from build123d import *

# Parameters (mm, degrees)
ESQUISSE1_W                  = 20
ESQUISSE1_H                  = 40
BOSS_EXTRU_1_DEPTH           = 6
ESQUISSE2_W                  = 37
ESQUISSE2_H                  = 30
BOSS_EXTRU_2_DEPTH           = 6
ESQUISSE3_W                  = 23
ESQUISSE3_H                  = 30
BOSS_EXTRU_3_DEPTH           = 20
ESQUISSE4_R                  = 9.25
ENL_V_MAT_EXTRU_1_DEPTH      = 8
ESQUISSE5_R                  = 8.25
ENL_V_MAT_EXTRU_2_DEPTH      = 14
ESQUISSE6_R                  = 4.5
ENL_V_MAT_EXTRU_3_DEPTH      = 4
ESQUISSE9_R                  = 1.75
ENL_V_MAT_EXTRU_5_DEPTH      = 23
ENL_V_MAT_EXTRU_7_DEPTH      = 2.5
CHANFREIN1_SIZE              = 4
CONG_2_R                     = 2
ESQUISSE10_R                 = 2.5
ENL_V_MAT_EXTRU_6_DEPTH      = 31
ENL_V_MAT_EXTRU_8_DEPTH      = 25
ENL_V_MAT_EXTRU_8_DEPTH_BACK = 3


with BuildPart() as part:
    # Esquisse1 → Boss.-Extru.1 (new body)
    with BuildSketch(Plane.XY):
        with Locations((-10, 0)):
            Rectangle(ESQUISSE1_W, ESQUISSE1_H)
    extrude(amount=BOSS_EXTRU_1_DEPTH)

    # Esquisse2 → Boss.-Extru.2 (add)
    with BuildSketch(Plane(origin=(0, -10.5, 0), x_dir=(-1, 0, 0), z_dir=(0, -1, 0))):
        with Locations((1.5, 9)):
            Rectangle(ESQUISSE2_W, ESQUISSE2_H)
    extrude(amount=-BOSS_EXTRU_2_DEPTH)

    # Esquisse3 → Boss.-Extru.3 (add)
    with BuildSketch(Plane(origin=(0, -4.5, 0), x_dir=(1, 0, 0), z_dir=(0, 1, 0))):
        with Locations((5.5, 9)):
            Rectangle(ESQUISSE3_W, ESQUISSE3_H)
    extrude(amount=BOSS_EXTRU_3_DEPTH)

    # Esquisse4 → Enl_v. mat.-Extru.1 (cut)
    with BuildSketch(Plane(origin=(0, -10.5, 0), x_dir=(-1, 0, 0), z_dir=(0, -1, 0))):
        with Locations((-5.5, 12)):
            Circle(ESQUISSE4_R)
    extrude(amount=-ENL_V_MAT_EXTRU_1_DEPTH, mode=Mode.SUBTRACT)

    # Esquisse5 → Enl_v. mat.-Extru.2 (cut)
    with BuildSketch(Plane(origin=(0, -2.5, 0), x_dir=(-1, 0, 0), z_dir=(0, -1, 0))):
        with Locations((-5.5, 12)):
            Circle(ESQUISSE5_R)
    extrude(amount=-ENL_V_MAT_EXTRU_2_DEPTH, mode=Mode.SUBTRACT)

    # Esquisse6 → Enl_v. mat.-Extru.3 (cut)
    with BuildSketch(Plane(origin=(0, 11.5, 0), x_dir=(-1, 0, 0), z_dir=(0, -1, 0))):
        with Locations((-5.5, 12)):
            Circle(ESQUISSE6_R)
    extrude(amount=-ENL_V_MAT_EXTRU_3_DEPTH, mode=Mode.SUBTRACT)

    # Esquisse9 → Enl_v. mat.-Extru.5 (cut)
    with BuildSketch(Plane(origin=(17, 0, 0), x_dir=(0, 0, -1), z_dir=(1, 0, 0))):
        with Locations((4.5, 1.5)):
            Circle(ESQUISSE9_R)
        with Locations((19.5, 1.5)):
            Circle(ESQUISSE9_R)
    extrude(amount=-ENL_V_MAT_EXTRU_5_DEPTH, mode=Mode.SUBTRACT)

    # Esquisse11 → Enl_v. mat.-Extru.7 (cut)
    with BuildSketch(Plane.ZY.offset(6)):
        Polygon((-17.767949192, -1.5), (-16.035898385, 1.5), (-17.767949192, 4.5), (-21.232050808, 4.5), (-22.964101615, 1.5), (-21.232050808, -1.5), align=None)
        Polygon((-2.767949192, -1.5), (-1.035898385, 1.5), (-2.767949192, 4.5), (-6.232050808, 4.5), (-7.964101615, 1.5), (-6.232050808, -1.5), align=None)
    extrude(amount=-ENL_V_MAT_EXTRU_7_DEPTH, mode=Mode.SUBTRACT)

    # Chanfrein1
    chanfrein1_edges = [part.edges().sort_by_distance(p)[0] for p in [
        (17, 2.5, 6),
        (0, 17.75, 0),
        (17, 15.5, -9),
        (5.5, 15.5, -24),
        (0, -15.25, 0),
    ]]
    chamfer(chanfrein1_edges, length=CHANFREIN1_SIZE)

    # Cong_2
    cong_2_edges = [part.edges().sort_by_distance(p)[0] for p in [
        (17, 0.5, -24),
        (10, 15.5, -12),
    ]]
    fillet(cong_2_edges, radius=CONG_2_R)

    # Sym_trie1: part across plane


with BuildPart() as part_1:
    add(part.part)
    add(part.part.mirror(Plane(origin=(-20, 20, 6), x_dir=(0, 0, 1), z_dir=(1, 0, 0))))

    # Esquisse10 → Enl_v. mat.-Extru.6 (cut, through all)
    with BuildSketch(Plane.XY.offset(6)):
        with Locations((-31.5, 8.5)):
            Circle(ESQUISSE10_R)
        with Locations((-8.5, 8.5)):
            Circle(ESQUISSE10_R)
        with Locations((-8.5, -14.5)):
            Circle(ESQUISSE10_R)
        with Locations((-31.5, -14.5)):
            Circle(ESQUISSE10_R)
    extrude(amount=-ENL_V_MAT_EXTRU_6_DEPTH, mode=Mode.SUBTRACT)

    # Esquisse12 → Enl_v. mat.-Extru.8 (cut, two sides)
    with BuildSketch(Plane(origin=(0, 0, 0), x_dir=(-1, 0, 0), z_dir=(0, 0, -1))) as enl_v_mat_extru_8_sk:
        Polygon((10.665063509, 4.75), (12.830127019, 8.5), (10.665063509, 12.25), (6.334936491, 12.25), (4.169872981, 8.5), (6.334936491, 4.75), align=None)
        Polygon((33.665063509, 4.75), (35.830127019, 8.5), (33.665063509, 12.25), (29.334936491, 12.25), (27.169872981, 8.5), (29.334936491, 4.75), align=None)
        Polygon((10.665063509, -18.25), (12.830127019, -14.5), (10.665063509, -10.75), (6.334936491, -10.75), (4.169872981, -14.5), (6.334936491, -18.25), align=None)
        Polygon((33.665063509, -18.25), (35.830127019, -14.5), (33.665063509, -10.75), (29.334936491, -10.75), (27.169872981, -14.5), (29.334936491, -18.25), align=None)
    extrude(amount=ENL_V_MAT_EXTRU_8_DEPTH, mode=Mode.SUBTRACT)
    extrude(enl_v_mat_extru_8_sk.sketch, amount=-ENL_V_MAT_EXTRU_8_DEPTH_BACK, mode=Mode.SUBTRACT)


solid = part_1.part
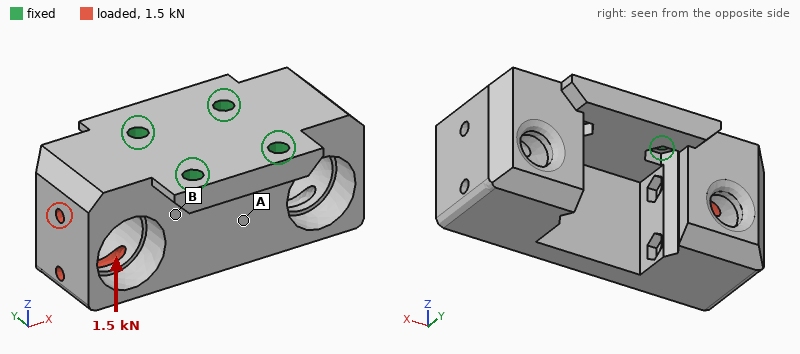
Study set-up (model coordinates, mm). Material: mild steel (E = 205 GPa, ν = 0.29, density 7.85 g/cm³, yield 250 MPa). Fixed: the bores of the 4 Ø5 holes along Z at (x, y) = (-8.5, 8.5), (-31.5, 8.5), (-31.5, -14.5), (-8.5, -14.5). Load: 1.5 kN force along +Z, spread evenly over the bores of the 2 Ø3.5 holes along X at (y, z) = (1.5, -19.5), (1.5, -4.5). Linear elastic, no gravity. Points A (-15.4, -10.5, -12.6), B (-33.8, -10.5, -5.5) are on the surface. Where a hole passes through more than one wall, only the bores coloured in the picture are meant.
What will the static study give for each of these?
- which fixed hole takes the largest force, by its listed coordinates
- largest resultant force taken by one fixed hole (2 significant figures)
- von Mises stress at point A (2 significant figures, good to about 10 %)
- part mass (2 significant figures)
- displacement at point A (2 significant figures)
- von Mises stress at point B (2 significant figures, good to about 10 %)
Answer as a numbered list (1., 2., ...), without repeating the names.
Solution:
1. (-31.5, 8.5)
2. 1.3 kN
3. 7.3 MPa
4. 260 g
5. 3.0 µm
6. 20 MPa
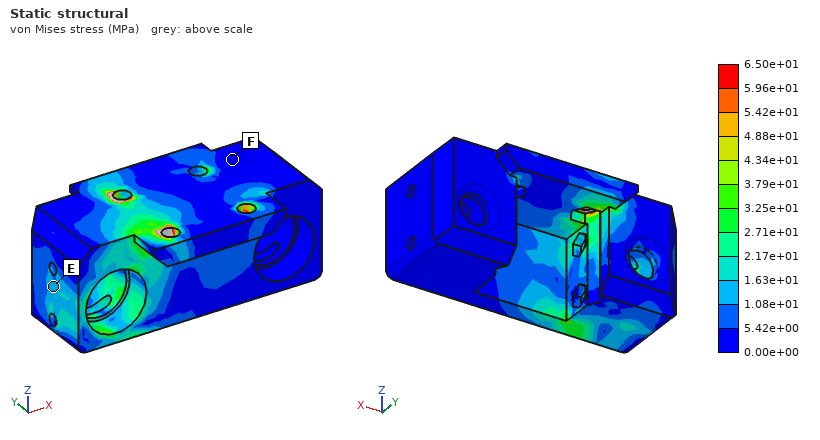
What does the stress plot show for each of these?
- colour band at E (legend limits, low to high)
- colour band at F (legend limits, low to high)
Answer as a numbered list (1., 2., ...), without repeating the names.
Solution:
1. 1.08e+01 to 1.63e+01 MPa
2. 0.00e+00 to 5.42e+00 MPa
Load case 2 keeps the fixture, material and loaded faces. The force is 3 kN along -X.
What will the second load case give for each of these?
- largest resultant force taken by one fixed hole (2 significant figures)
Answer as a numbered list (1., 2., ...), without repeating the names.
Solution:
1. 1.6 kN
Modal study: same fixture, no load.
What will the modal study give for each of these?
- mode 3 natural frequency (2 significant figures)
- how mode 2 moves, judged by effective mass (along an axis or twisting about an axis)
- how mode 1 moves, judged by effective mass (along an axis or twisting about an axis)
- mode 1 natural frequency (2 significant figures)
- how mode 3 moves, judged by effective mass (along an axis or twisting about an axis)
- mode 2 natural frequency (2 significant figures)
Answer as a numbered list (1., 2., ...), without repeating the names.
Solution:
1. 8000 Hz
2. along Z
3. along X
4. 5000 Hz
5. along Y
6. 7400 Hz
